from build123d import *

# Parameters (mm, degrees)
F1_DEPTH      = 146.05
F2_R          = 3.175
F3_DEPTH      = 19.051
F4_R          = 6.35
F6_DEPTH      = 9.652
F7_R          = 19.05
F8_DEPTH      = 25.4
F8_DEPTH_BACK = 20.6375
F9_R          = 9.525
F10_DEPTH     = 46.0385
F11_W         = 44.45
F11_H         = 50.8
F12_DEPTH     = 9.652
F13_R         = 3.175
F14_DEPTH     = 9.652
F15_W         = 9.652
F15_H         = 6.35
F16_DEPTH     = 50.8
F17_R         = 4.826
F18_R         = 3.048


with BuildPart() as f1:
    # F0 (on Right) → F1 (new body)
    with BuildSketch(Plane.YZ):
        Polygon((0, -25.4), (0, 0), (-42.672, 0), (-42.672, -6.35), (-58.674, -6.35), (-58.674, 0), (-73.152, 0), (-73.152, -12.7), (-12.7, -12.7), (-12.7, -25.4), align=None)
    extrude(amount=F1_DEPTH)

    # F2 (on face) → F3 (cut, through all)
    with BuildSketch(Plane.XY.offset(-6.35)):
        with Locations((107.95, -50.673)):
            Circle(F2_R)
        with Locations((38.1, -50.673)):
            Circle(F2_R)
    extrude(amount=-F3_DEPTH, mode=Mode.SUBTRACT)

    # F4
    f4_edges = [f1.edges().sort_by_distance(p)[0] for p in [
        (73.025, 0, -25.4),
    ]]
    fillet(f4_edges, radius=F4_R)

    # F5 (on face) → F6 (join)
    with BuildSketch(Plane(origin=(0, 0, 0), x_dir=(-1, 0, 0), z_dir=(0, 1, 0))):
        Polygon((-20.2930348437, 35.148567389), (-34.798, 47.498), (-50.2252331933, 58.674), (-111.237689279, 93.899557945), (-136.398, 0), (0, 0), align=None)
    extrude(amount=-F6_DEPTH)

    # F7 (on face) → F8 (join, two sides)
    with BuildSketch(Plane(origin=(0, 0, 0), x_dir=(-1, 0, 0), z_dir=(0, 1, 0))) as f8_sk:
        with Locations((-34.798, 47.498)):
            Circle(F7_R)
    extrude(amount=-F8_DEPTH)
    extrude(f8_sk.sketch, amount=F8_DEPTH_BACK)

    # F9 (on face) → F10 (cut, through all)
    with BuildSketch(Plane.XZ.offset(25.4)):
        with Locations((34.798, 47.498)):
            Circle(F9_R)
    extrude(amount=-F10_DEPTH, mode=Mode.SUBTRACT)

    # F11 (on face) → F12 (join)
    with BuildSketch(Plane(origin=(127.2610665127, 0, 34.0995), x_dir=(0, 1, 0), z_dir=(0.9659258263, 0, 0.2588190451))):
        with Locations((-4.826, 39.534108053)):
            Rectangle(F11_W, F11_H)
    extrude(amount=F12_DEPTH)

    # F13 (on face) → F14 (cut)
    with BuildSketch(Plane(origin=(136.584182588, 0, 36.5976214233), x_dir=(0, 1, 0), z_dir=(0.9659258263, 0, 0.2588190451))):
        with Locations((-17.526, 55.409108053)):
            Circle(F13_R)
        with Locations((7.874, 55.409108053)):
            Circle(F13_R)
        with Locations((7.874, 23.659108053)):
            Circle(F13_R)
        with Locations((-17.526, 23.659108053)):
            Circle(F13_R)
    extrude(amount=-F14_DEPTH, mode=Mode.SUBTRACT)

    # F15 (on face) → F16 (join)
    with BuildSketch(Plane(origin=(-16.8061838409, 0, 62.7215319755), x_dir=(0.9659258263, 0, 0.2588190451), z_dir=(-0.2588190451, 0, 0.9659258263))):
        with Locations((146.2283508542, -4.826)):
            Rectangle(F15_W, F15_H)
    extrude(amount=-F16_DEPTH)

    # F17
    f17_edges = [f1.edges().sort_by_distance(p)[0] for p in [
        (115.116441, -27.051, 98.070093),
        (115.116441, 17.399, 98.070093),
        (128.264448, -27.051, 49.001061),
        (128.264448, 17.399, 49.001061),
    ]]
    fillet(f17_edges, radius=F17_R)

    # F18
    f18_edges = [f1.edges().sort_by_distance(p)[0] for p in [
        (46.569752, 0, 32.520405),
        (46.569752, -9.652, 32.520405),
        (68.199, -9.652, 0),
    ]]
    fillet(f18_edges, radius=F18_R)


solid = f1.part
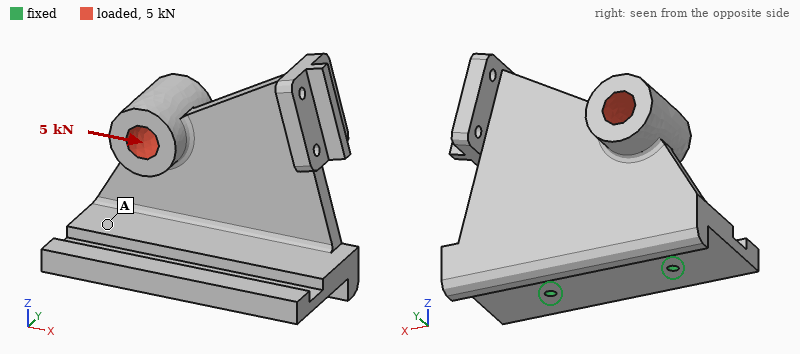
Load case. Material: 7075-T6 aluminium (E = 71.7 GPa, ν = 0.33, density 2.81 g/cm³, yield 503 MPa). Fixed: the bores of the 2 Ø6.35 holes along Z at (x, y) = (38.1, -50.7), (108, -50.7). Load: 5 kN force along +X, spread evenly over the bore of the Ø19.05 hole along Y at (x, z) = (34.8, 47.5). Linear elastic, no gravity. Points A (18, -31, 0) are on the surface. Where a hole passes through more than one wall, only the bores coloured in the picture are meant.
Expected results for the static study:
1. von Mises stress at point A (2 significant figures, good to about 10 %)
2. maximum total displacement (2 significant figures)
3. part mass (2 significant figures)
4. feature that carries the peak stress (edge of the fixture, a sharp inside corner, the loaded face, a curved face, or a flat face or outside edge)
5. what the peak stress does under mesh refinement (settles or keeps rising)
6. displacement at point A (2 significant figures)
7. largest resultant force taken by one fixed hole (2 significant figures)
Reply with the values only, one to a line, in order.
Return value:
17 MPa
0.47 mm
770 g
edge of the fixture
keeps rising
0.12 mm
5.6 kN
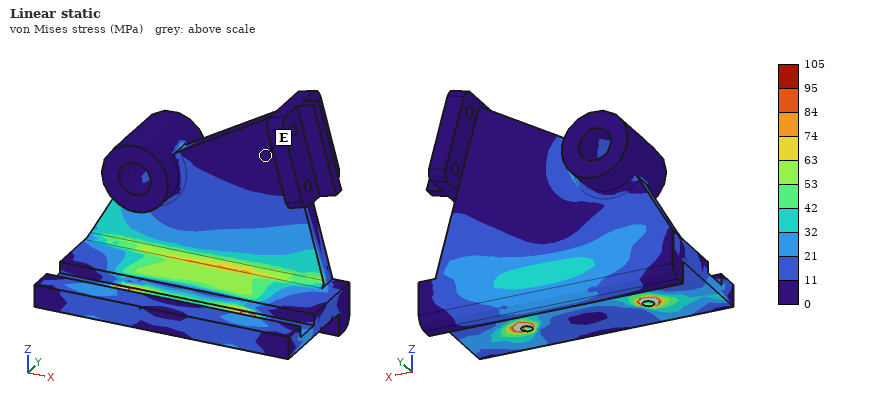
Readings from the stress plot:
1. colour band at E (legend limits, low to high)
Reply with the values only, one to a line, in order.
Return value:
0 to 11 MPa
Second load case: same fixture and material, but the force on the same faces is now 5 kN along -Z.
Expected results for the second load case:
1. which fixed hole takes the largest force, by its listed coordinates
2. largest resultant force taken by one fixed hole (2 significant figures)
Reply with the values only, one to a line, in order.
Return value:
(38.1, -50.7)
5.0 kN
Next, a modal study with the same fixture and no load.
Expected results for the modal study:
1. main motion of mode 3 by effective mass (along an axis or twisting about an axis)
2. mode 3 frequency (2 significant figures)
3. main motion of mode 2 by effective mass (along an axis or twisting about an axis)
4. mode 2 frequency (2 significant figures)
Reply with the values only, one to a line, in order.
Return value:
along Z
1100 Hz
along X
890 Hz
